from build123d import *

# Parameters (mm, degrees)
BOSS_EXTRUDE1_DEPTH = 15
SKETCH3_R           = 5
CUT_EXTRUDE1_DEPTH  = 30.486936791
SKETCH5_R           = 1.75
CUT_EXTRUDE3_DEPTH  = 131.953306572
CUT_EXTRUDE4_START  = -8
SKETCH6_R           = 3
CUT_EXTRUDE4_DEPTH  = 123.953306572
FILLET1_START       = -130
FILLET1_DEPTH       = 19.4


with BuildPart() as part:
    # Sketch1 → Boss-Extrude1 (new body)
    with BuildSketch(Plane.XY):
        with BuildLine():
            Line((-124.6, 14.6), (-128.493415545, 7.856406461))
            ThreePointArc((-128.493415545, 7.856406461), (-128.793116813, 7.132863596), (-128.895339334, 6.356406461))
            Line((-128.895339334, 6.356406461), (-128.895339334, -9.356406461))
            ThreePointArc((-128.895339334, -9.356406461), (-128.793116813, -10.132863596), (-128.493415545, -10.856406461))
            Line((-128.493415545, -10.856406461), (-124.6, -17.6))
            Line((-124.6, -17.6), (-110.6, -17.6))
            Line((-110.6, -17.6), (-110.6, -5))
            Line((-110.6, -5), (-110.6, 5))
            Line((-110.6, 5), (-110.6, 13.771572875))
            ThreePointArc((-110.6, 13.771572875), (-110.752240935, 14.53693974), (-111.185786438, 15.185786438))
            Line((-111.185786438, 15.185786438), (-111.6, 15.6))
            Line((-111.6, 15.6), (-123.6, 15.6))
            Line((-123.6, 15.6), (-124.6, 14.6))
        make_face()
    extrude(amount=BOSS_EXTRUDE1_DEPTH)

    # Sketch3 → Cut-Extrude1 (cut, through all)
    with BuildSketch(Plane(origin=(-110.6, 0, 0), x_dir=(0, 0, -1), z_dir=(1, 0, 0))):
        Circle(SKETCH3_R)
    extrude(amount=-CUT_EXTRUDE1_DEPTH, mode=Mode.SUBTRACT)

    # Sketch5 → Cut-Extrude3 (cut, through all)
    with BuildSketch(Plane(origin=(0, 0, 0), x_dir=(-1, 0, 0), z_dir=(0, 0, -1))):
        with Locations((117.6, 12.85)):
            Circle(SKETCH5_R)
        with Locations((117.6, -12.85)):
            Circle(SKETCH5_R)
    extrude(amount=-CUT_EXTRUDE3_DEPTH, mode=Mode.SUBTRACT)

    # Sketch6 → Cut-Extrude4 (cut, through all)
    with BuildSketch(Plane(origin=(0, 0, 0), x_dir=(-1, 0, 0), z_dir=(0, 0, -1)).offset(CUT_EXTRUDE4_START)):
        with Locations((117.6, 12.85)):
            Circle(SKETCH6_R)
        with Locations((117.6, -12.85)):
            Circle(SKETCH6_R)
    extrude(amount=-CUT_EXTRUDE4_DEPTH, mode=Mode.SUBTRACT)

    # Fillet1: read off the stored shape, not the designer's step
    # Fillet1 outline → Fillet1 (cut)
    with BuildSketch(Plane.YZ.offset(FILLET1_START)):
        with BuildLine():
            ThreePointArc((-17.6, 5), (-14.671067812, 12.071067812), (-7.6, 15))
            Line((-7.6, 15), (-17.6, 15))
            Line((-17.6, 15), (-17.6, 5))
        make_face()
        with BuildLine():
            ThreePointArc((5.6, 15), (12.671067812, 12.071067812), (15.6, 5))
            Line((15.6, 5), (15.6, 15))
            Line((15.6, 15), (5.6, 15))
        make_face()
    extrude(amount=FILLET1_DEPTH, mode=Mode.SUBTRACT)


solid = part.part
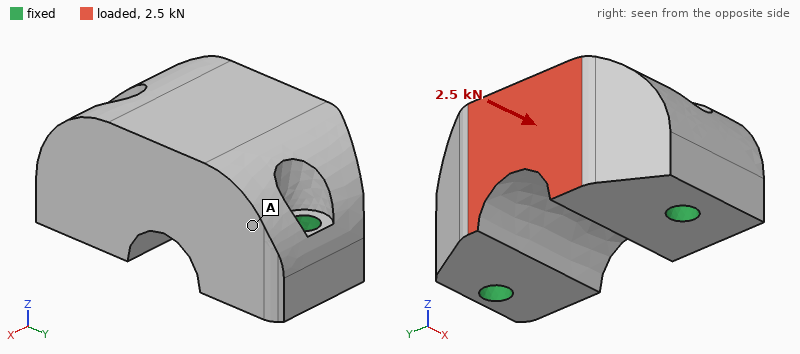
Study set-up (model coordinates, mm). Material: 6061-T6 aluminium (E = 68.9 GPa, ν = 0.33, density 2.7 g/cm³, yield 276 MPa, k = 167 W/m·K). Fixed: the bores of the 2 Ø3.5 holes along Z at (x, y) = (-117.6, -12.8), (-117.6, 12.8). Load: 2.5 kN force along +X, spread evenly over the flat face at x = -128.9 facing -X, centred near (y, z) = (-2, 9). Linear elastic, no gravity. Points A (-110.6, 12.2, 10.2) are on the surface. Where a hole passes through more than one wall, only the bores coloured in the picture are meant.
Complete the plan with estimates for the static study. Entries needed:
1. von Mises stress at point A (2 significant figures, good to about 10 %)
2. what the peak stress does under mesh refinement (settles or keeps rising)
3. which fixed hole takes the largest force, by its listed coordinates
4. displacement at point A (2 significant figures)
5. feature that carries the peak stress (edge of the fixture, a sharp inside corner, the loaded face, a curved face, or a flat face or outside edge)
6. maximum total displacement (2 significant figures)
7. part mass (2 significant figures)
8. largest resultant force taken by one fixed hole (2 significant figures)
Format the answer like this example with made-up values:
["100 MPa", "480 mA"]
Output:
["8.3 MPa", "keeps rising", "(-117.6, -12.8)", "5.3 µm", "edge of the fixture", "14 µm", "18 g", "1.5 kN"]
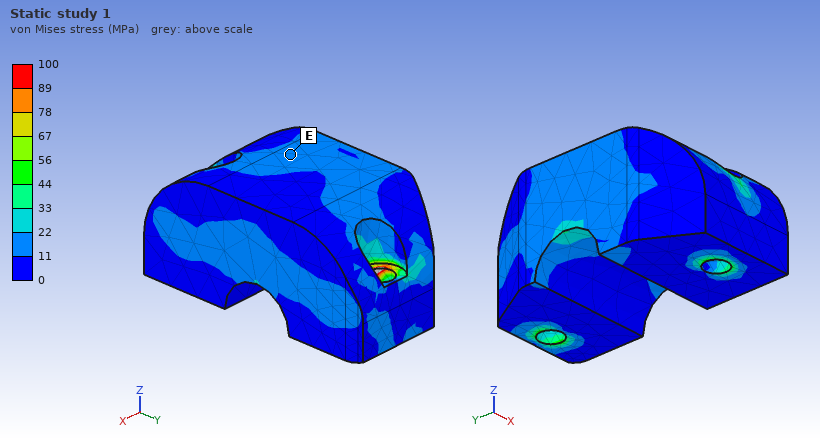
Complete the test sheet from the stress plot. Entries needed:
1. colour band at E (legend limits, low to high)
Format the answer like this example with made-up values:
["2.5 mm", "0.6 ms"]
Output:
["11 to 22 MPa"]
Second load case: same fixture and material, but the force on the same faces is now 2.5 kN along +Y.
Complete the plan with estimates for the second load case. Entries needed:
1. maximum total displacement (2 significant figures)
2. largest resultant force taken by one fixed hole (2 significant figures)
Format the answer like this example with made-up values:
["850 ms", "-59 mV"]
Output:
["7.8 µm", "1.7 kN"]
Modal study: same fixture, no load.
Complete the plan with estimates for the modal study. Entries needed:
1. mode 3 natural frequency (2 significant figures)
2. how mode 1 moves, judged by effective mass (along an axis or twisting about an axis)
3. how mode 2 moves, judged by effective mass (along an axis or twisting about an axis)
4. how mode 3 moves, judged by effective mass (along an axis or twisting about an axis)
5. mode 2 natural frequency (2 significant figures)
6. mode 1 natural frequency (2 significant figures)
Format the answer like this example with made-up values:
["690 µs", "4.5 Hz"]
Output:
["44 kHz", "along X", "along Z", "along Y", "37 kHz", "21 kHz"]
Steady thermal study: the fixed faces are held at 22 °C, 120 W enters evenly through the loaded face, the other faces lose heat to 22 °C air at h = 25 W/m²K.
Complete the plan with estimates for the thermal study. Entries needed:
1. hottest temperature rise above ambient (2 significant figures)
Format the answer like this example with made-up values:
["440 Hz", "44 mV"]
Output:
["44 K"]
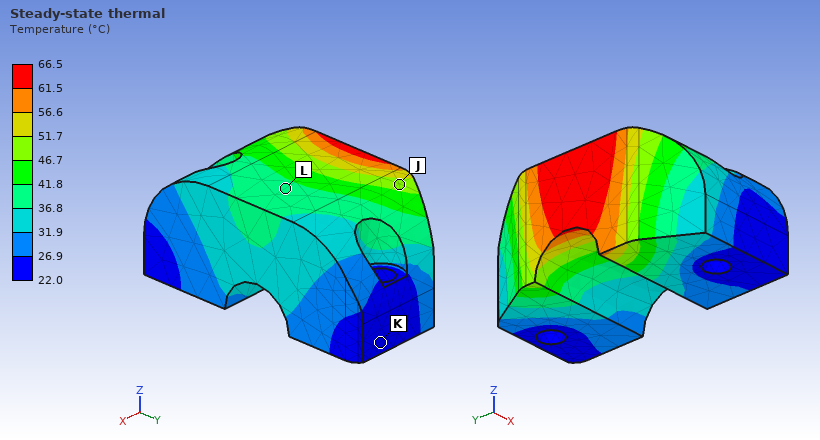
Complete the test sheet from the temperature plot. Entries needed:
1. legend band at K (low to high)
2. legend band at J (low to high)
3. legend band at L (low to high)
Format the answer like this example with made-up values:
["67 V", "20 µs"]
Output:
["22.0 to 26.9 °C", "46.7 to 51.7 °C", "36.8 to 41.8 °C"]
